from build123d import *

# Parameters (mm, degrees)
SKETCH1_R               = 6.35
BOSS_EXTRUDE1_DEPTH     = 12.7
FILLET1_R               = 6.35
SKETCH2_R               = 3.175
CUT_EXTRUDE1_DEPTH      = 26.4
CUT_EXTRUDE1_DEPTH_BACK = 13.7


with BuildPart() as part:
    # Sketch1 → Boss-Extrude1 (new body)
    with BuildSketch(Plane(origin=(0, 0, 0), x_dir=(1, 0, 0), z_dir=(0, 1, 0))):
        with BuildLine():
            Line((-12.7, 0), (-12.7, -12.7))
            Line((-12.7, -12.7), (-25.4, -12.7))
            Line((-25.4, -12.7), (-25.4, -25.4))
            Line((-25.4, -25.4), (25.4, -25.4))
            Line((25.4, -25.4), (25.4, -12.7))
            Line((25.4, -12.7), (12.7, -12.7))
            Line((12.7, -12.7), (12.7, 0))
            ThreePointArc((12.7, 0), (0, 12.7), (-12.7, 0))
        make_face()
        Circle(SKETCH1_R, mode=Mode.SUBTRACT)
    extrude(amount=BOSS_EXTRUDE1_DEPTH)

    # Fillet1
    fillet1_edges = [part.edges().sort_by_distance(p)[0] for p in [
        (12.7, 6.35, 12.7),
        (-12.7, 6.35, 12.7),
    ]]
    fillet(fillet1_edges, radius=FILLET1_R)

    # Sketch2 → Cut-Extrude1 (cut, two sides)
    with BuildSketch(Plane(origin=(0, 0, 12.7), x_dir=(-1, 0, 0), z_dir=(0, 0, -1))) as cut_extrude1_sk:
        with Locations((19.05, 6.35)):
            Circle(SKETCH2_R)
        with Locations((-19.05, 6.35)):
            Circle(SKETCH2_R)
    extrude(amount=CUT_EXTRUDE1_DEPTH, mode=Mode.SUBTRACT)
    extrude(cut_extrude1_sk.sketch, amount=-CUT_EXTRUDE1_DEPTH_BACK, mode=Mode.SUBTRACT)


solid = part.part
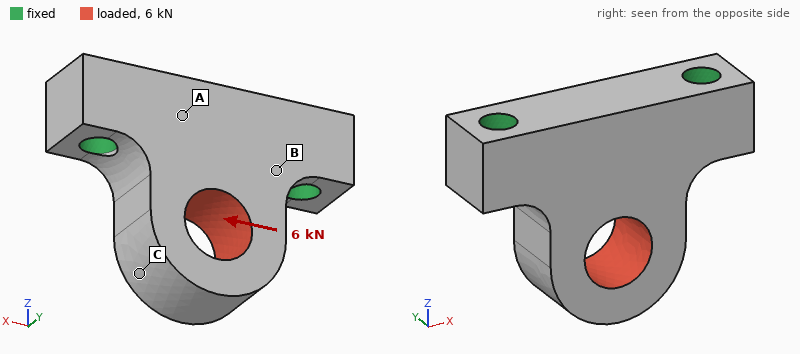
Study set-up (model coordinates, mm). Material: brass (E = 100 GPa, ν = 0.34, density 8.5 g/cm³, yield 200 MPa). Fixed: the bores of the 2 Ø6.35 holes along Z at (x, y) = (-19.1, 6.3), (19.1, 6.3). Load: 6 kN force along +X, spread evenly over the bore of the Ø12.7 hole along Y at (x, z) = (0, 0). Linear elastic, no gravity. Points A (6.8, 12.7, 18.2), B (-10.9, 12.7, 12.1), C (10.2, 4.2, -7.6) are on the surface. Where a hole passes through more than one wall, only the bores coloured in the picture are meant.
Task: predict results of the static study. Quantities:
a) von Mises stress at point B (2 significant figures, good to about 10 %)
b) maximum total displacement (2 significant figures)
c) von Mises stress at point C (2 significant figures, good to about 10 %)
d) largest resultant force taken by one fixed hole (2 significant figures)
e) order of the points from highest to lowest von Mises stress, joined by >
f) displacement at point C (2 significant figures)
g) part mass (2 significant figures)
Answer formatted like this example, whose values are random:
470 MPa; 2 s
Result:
20 MPa; 32 µm; 34 MPa; 4.3 kN; C > B > A; 31 µm; 110 g
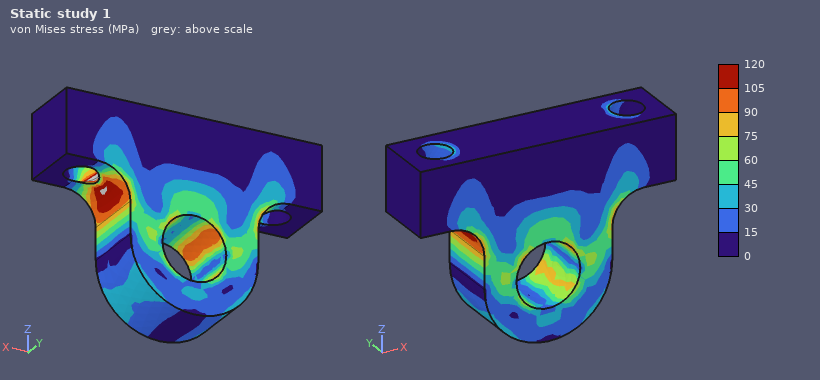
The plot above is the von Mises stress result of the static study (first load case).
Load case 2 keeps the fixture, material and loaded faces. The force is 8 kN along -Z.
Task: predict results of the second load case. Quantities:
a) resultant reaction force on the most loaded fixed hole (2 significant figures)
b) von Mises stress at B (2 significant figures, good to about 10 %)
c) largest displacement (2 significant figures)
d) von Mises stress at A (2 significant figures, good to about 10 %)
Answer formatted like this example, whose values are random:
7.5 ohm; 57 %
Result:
4.3 kN; 25 MPa; 14 µm; 16 MPa
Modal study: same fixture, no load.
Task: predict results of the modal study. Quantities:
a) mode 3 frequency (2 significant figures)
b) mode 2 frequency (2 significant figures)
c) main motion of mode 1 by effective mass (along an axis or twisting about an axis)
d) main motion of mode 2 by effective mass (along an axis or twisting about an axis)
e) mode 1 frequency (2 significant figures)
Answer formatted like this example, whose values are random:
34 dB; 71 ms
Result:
15 kHz; 12 kHz; along Y; along X; 6100 Hz
